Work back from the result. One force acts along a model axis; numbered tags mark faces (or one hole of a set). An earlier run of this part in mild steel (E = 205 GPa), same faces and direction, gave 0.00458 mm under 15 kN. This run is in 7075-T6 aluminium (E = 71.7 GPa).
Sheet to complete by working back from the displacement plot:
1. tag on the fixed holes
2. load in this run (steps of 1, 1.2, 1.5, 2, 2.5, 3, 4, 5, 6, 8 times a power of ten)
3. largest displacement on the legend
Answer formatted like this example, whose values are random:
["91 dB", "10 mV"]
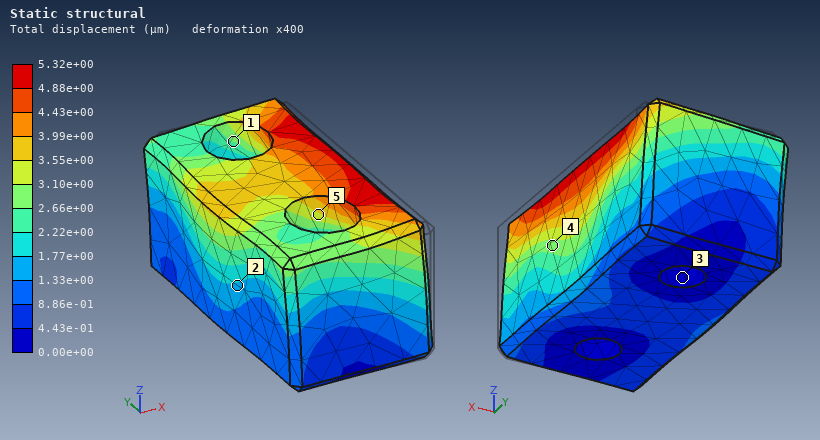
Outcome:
["3", "6 kN", "5.32e+00 µm"]
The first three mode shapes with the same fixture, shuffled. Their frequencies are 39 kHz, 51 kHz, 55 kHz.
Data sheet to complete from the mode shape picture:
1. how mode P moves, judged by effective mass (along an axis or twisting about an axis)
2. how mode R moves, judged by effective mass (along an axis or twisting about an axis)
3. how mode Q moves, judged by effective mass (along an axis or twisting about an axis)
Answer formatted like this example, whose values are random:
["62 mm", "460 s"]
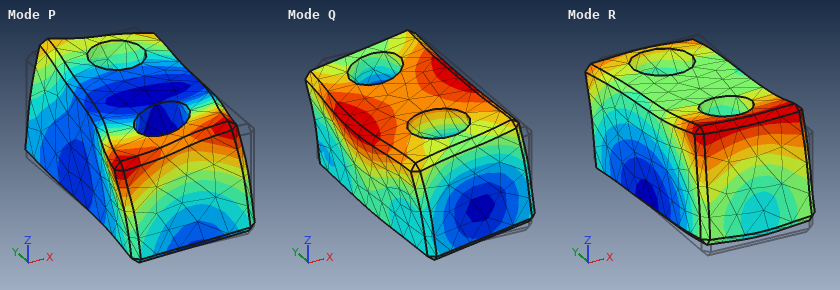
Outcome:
["twisting about Z", "along Y", "along X"]
